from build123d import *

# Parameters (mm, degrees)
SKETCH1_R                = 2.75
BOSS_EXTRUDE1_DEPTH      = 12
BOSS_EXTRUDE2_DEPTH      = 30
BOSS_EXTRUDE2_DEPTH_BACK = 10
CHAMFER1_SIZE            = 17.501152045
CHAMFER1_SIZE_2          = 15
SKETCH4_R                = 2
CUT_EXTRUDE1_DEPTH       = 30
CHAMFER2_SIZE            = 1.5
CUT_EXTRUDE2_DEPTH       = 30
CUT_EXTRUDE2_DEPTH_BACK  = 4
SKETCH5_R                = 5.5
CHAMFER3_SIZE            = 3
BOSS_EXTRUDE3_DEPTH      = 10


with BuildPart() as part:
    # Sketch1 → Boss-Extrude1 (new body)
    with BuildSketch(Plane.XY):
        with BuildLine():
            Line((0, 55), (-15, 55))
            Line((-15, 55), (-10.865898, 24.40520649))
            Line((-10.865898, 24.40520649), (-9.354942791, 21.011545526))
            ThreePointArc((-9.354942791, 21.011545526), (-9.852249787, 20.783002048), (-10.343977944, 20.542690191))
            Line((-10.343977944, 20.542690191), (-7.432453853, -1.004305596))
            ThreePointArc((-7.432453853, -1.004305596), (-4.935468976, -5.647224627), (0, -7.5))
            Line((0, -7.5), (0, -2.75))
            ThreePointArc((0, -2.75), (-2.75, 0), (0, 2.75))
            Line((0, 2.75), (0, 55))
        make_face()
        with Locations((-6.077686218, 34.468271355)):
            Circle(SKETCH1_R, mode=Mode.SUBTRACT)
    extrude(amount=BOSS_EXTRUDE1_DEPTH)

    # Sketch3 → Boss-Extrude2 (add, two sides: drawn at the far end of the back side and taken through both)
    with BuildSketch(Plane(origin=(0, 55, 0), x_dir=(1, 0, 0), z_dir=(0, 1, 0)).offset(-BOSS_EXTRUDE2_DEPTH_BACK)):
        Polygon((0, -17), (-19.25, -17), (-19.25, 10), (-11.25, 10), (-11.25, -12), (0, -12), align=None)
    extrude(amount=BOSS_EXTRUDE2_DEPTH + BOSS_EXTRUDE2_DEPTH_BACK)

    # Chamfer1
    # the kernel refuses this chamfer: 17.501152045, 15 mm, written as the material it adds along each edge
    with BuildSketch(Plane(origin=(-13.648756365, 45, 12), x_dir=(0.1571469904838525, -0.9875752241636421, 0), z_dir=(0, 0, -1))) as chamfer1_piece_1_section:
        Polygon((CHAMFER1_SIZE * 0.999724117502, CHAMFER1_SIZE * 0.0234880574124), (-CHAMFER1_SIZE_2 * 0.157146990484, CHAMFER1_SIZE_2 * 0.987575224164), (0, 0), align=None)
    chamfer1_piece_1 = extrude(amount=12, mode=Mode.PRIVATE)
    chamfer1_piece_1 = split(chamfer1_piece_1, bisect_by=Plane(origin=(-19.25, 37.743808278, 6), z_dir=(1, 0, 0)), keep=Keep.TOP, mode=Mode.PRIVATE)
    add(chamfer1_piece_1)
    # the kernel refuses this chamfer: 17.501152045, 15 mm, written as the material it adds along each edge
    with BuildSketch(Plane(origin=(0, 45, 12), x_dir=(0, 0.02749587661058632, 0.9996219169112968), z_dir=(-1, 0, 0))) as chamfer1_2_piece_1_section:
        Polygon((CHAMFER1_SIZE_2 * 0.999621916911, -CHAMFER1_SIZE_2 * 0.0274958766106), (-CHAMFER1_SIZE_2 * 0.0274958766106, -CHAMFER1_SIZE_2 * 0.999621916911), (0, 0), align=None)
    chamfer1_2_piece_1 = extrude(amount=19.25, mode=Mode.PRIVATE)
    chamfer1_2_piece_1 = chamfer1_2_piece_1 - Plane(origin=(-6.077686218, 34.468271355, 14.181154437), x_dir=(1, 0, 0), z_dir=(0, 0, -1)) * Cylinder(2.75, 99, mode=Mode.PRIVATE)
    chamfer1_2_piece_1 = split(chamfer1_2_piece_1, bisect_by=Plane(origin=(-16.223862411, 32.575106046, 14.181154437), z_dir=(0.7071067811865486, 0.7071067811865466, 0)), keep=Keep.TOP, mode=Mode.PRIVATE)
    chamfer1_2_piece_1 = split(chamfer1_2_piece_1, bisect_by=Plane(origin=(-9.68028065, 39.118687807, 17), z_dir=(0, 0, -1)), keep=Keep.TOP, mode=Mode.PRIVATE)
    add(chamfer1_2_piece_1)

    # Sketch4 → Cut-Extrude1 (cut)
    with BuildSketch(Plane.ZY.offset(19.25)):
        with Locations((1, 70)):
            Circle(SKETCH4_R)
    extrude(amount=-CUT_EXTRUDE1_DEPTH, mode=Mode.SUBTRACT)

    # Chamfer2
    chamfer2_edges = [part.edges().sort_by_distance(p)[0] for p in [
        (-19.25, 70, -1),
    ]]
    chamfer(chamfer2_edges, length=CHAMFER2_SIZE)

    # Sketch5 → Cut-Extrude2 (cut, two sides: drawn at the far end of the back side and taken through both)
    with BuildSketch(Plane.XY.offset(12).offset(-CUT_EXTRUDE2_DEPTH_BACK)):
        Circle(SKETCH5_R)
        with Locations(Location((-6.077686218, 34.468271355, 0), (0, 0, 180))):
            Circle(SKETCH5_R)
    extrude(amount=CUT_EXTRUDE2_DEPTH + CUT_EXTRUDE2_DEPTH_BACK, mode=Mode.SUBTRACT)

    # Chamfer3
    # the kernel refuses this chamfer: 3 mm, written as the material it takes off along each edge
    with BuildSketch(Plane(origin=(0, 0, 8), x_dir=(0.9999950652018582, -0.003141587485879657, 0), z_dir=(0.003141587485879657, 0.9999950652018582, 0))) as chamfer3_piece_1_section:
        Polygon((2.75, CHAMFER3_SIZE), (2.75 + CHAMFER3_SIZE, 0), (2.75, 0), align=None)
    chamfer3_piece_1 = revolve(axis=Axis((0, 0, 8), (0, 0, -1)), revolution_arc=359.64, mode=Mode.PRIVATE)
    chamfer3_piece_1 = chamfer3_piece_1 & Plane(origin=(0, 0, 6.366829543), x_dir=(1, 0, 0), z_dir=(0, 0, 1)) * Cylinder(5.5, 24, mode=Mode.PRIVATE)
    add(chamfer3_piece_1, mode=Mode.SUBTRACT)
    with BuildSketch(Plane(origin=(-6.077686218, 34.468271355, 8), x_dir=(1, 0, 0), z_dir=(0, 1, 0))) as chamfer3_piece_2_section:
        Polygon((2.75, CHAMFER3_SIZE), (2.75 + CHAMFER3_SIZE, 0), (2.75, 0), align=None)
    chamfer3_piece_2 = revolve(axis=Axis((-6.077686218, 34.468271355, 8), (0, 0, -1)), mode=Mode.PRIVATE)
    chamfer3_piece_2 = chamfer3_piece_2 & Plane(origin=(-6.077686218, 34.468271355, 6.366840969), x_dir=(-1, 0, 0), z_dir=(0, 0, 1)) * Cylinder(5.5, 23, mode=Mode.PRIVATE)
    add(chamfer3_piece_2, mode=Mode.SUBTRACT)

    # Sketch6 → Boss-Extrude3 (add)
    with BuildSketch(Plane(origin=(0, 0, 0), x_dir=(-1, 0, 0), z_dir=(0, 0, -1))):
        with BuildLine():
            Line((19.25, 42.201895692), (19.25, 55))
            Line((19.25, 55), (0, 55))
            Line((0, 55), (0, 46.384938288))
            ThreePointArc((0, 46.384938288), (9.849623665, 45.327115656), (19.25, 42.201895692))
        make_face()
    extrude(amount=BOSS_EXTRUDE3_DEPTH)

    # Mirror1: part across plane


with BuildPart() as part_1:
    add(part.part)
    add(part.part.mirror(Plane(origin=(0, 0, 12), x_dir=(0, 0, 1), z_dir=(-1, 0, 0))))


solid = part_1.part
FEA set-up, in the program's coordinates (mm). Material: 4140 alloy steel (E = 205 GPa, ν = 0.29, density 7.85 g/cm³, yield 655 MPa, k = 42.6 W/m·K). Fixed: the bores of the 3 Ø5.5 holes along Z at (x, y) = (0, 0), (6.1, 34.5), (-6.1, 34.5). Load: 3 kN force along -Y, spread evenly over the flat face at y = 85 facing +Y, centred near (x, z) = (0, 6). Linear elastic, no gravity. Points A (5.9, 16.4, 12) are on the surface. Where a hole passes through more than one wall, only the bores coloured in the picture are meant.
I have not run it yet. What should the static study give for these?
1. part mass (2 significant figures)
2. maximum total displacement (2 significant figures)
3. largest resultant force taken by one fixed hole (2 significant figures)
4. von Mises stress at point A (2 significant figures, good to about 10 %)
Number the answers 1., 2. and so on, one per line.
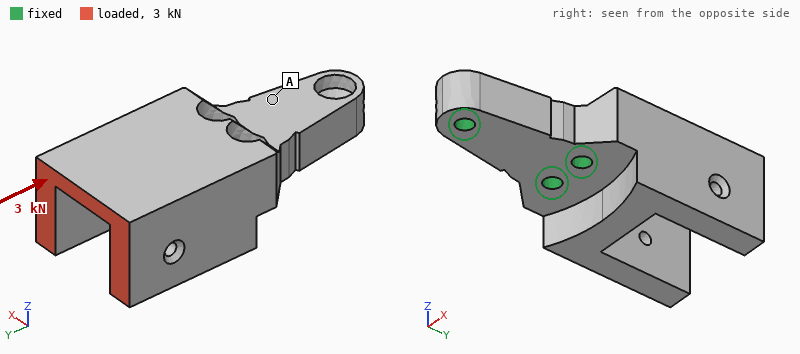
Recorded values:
1. 320 g
2. 4.7 µm
3. 1.3 kN
4. 4.0 MPa
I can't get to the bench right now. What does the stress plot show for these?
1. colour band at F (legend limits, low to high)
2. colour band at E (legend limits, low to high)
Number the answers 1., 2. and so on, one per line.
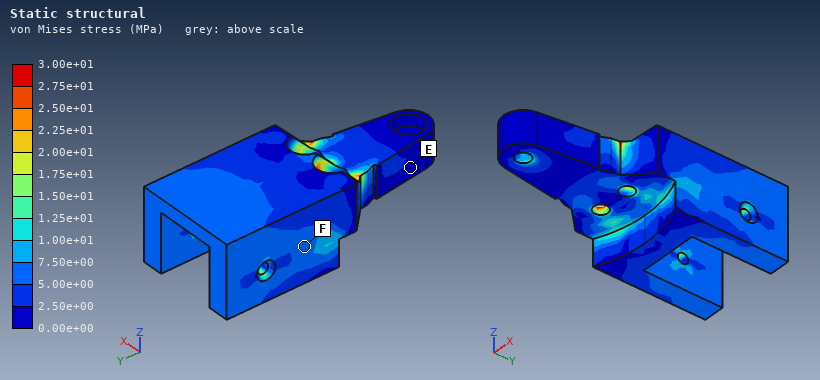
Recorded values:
1. 5.00e+00 to 7.50e+00 MPa
2. 0.00e+00 to 2.50e+00 MPa
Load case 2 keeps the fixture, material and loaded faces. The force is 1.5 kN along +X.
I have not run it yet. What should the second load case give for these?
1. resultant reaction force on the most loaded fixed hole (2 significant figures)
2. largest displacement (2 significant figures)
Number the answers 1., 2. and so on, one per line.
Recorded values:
1. 3.5 kN
2. 32 µm
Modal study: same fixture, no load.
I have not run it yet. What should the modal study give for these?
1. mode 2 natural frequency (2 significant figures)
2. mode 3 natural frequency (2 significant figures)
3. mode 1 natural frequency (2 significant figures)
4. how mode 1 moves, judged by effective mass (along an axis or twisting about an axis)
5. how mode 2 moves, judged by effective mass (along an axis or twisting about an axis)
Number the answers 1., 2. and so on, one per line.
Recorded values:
1. 4700 Hz
2. 5900 Hz
3. 2700 Hz
4. along Z
5. along X
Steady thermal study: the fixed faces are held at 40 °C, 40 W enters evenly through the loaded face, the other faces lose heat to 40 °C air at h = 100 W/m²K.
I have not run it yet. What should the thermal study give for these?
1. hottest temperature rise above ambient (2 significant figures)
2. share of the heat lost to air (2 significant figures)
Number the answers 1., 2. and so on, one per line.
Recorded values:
1. 58 K
2. 62 %
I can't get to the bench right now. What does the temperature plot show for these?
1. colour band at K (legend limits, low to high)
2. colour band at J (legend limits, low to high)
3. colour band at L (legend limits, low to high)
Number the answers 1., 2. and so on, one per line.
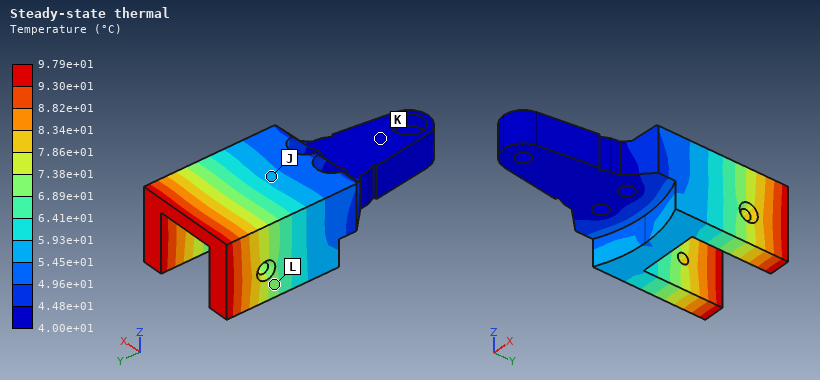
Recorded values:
1. 4.00e+01 to 4.48e+01 °C
2. 5.45e+01 to 5.93e+01 °C
3. 6.89e+01 to 7.38e+01 °C
